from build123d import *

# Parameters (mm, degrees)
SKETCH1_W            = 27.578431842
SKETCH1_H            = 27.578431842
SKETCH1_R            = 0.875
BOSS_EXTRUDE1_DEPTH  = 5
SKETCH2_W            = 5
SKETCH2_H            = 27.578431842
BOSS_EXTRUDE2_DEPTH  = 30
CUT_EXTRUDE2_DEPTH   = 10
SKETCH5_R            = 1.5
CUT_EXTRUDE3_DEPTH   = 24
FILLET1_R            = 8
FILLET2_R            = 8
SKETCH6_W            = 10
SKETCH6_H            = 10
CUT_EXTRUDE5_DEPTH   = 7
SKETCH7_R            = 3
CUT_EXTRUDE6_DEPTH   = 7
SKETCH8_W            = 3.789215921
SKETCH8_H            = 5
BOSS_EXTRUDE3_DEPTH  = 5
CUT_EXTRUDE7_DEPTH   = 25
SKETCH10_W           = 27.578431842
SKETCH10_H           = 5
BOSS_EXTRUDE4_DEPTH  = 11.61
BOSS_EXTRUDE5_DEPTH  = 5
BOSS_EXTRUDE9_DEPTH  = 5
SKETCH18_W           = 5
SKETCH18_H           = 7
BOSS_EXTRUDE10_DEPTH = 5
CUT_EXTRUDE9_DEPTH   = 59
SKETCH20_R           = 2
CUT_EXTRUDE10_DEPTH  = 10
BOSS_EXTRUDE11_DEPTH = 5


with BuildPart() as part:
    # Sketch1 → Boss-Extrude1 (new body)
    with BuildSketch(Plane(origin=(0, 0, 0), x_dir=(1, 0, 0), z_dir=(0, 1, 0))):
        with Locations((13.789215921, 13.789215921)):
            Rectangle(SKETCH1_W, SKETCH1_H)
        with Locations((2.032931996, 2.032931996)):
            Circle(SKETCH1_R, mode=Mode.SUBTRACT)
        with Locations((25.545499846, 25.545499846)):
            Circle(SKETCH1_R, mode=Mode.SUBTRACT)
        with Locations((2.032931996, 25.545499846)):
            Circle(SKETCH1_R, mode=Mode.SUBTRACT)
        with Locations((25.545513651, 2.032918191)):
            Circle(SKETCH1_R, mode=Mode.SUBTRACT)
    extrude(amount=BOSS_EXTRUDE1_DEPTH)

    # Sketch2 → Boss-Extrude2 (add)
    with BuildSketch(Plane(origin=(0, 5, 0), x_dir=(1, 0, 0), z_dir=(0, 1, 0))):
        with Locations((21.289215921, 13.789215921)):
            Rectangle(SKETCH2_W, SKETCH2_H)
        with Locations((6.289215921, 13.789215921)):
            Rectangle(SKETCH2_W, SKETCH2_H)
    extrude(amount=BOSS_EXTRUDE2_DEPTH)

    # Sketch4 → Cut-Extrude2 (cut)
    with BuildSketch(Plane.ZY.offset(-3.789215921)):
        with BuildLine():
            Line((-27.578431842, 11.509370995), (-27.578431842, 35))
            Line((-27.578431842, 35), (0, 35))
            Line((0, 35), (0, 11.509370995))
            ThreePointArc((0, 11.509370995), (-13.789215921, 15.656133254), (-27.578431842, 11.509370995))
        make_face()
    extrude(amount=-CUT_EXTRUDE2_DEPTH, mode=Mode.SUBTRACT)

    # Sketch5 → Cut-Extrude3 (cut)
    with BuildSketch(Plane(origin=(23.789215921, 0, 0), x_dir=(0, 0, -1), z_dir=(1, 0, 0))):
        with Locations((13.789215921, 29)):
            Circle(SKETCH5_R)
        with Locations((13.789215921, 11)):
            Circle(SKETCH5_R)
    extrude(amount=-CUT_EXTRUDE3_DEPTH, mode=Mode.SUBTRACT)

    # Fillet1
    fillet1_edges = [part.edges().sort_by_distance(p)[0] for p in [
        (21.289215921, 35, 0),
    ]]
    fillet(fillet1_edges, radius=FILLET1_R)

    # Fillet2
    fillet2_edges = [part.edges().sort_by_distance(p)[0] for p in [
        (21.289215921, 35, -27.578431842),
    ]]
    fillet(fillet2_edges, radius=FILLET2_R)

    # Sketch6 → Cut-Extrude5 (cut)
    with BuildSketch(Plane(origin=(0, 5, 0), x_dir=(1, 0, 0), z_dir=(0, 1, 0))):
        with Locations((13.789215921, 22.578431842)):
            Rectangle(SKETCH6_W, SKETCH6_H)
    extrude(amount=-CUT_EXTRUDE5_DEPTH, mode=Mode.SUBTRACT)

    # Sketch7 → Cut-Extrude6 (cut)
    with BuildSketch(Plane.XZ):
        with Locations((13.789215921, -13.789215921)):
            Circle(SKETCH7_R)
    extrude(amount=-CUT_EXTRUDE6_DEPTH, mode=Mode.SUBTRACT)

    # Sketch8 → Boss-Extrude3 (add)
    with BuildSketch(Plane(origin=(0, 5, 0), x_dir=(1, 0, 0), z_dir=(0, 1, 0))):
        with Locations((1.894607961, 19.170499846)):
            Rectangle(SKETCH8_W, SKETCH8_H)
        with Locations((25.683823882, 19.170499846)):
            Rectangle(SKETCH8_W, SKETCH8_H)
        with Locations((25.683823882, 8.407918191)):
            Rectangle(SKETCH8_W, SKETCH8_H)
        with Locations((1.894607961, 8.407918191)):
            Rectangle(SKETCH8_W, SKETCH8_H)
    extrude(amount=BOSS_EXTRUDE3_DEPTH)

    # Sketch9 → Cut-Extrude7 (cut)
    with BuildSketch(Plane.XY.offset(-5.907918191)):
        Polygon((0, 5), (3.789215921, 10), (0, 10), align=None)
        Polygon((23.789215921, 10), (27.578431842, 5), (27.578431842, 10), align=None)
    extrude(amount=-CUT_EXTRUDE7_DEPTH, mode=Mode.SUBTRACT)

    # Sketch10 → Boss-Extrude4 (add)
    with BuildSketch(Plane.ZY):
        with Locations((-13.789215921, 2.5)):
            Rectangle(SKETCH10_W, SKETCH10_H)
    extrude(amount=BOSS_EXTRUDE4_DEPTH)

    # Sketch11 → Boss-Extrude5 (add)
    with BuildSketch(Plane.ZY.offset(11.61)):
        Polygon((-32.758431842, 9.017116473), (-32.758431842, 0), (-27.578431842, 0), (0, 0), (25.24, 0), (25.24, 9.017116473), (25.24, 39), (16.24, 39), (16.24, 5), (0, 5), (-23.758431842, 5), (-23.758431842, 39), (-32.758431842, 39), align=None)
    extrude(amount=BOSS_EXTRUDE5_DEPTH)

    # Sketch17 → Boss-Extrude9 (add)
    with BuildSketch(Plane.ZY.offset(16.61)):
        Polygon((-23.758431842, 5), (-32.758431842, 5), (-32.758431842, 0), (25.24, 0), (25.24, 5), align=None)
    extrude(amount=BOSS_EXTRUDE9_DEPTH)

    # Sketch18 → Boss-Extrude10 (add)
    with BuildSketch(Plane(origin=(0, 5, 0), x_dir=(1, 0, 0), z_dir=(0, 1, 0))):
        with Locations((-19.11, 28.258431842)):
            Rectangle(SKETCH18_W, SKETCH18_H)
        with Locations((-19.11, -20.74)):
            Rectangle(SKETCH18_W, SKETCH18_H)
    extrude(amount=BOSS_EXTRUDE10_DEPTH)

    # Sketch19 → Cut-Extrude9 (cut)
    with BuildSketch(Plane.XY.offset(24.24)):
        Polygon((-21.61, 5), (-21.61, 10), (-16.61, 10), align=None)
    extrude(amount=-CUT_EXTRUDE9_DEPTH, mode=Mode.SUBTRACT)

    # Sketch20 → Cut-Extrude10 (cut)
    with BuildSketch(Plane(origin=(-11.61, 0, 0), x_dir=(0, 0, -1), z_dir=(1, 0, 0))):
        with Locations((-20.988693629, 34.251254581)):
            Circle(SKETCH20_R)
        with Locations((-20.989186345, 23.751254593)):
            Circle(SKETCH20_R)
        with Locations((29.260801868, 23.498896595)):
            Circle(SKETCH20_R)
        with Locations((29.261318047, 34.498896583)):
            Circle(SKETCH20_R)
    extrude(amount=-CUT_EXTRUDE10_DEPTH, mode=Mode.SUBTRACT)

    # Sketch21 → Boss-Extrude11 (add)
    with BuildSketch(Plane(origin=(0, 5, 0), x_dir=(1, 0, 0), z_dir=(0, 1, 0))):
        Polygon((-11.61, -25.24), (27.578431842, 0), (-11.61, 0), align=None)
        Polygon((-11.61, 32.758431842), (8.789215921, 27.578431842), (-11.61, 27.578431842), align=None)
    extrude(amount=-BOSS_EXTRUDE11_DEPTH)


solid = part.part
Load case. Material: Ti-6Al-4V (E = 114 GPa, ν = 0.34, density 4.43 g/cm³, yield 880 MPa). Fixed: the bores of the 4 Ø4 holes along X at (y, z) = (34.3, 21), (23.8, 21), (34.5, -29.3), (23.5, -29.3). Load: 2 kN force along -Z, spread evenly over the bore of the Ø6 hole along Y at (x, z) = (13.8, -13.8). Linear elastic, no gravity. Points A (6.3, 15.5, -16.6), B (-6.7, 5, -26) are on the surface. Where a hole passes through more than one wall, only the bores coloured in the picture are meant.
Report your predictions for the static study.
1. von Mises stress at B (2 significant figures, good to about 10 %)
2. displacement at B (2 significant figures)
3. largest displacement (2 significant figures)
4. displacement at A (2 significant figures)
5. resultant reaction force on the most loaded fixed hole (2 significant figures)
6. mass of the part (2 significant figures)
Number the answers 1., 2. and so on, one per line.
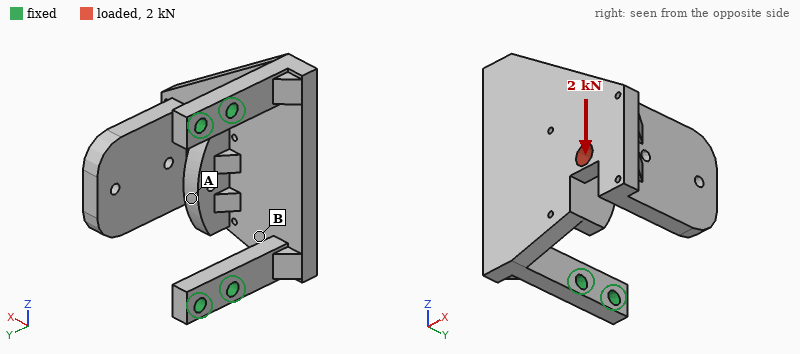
1. 120 MPa
2. 0.12 mm
3. 0.33 mm
4. 0.18 mm
5. 1.9 kN
6. 83 g
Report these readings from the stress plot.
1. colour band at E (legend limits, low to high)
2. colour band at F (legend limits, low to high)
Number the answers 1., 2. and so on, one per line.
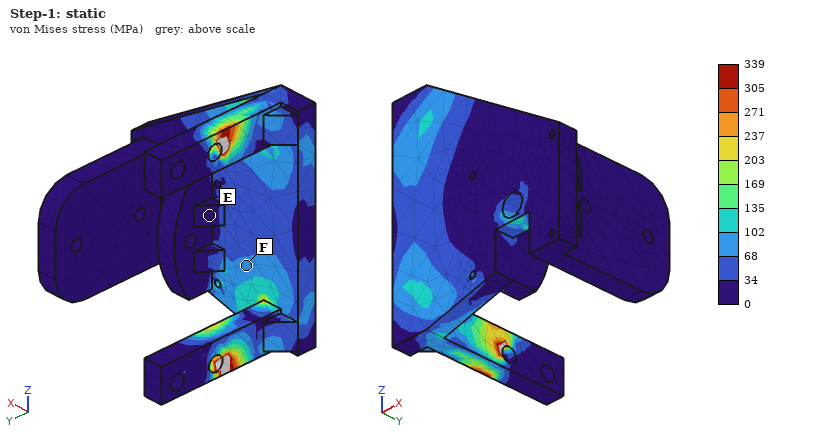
1. 0 to 34 MPa
2. 68 to 102 MPa
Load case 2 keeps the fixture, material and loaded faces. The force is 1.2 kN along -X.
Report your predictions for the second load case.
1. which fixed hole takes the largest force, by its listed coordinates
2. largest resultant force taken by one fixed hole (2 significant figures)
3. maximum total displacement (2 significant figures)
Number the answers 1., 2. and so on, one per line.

1. (23.5, -29.3)
2. 930 N
3. 0.51 mm
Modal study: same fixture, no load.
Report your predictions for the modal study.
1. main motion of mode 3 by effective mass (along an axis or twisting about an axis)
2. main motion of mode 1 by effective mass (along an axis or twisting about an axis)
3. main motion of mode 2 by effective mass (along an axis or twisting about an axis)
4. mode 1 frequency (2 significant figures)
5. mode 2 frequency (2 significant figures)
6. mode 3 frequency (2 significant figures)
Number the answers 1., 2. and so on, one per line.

1. along X
2. along Y
3. along Z
4. 710 Hz
5. 1700 Hz
6. 1900 Hz
